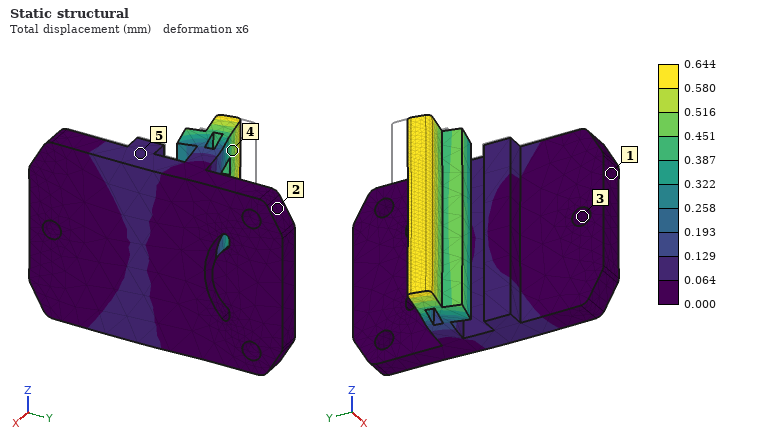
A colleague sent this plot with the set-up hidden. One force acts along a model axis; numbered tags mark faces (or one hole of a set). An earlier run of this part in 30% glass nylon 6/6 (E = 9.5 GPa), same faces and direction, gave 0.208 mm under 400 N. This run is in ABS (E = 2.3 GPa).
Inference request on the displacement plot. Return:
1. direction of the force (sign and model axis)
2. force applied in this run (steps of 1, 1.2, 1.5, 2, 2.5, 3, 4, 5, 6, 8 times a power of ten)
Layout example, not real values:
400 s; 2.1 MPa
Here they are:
-Y; 300 N
